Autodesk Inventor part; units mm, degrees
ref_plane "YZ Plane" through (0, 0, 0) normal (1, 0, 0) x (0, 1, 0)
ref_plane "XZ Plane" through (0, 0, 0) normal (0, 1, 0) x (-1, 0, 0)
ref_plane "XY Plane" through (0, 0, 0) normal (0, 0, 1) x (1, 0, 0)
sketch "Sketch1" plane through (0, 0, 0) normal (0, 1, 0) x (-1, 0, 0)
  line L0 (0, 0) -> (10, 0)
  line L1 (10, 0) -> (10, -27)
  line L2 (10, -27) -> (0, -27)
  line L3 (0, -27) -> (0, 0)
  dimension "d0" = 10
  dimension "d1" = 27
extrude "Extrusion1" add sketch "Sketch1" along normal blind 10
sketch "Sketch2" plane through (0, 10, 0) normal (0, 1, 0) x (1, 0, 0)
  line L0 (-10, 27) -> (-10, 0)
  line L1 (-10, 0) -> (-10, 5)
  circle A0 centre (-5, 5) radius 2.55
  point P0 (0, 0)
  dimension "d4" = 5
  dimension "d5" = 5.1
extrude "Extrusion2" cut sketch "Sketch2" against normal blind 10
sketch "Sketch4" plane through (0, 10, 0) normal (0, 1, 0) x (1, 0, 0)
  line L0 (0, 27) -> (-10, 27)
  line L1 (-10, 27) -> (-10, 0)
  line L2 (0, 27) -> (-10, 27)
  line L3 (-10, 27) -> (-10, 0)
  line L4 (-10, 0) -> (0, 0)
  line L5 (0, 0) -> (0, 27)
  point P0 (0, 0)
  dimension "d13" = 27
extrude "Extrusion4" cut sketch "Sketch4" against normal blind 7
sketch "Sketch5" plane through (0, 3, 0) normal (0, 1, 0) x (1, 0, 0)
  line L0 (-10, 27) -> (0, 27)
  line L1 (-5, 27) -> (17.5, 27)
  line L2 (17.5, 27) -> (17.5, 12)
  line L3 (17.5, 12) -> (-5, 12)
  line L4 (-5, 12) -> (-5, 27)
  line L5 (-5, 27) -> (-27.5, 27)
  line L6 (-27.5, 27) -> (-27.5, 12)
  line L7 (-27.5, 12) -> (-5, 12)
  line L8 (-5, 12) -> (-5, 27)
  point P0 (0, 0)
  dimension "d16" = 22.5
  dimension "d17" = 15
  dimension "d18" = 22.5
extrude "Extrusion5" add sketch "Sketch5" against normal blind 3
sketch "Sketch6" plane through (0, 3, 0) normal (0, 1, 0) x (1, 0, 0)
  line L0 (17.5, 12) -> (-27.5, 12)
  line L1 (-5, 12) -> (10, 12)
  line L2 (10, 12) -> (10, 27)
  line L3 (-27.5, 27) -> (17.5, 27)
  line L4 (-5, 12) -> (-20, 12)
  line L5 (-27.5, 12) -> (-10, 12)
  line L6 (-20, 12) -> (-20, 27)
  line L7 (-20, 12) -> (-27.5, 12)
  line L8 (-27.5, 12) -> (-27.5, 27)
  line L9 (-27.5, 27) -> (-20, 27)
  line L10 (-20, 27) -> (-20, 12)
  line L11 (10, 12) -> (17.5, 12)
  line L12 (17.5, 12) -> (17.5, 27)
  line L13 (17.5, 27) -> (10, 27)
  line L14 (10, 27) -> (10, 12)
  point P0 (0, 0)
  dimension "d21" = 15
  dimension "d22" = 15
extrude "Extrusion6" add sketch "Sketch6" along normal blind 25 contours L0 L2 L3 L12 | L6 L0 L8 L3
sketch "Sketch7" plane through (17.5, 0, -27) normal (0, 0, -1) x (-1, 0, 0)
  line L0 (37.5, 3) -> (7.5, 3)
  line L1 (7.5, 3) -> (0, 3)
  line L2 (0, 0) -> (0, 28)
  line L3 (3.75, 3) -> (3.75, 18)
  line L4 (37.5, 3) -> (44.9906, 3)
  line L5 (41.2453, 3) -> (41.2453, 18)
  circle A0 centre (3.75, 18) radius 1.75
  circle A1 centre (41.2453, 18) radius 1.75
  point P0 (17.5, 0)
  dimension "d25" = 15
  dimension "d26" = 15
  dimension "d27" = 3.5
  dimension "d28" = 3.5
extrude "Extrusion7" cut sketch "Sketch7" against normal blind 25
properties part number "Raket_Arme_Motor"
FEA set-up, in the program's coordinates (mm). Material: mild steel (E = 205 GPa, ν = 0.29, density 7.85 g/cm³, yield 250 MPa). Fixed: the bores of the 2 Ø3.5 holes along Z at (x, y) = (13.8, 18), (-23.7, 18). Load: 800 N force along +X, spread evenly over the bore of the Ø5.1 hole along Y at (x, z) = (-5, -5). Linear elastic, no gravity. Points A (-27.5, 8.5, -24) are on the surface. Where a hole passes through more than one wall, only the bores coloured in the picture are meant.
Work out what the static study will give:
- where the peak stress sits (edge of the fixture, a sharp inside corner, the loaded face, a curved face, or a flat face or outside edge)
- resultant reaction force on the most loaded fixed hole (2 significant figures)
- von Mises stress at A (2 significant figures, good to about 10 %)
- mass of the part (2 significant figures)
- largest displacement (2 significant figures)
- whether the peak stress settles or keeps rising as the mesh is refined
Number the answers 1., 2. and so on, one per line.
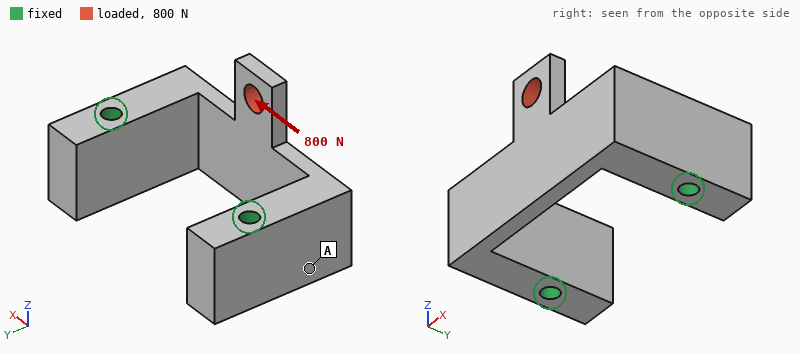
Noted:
1. a sharp inside corner
2. 510 N
3. 18 MPa
4. 60 g
5. 29 µm
6. keeps rising
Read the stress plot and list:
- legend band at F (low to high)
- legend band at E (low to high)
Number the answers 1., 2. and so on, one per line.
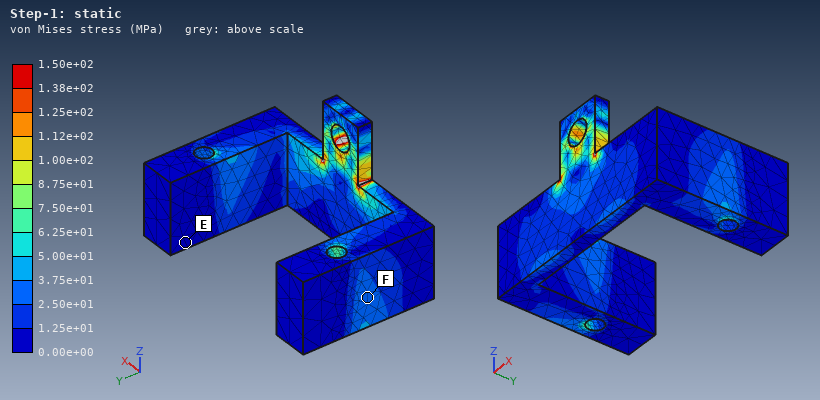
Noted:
1. 2.50e+01 to 3.75e+01 MPa
2. 0.00e+00 to 1.25e+01 MPa
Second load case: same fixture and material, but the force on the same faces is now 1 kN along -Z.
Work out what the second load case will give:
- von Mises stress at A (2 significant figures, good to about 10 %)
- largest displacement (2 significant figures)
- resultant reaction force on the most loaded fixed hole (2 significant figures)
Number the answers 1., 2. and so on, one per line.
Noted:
1. 8.6 MPa
2. 11 µm
3. 500 N
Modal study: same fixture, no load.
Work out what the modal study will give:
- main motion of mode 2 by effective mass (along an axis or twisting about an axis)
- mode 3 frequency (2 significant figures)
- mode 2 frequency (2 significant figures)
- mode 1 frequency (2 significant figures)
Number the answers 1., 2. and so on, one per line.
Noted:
1. along X
2. 14 kHz
3. 11 kHz
4. 6900 Hz
